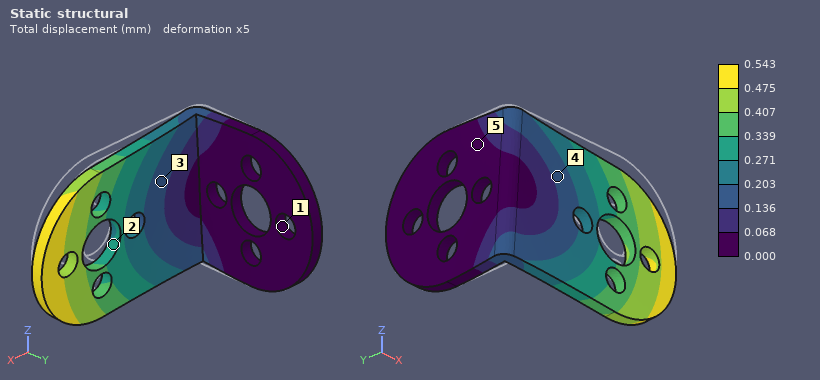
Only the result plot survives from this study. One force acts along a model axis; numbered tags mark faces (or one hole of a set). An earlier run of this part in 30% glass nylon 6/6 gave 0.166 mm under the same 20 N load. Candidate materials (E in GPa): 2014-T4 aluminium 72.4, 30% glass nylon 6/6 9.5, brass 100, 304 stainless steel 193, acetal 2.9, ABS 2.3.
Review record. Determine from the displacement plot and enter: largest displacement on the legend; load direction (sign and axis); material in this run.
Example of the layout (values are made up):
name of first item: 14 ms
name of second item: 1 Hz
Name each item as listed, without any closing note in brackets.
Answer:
largest displacement on the legend: 0.543 mm
load direction: -Z
material in this run: acetal
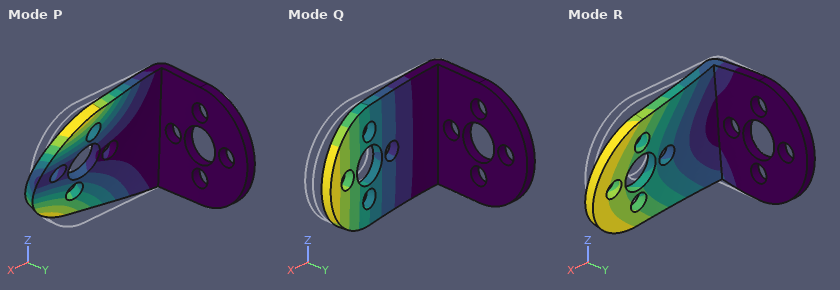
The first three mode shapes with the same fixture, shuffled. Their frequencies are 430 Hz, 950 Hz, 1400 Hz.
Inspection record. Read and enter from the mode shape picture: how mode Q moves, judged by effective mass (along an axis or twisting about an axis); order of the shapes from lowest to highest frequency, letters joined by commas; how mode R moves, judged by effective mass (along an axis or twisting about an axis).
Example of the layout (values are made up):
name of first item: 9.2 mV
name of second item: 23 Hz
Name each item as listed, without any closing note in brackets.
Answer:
how mode Q moves, judged by effective mass: along Y
order of the shapes from lowest to highest frequency, letters joined by commas: Q, R, P
how mode R moves, judged by effective mass: along Z
